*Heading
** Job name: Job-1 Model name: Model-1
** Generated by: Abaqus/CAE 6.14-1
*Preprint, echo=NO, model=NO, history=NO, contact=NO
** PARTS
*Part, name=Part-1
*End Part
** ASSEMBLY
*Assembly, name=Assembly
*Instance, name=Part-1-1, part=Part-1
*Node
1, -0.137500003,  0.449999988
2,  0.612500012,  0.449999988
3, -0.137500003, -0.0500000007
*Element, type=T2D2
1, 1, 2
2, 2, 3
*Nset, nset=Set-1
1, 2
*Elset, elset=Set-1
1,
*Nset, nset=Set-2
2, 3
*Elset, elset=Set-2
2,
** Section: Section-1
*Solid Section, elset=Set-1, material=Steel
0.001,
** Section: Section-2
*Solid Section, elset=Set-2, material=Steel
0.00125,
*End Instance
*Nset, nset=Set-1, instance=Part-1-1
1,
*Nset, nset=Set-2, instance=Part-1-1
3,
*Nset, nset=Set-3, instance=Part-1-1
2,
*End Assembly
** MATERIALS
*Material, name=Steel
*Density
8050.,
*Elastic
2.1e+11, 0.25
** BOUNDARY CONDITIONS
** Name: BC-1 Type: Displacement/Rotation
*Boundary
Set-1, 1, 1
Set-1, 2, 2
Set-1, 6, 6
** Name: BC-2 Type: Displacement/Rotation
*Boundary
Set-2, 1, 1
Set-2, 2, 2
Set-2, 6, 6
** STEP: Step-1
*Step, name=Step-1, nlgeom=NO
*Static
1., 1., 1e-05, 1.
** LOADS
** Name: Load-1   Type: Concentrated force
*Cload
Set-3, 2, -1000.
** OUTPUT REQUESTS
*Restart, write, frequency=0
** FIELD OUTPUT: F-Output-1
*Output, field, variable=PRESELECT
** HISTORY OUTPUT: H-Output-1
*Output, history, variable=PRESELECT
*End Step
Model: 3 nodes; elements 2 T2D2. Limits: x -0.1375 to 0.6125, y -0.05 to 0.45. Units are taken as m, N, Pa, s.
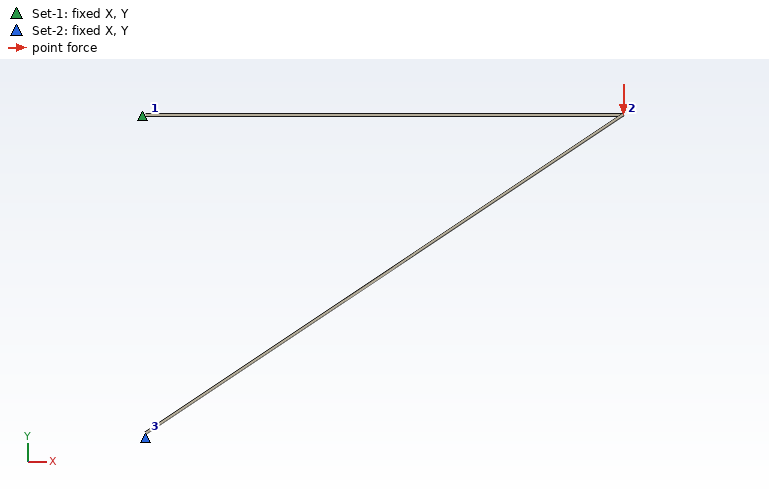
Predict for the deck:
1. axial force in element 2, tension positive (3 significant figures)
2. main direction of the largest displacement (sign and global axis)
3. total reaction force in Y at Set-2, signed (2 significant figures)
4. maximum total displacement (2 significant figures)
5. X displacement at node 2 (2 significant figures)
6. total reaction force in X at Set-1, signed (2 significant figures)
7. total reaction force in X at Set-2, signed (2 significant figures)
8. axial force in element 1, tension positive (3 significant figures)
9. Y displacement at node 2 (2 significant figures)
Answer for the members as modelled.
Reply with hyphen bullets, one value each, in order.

- -1800 N
- -Y
- 1000 N
- 2.0e-05 m
- 5.4e-06 m
- -1500 N
- 1500 N
- 1500 N
- -1.9e-05 m
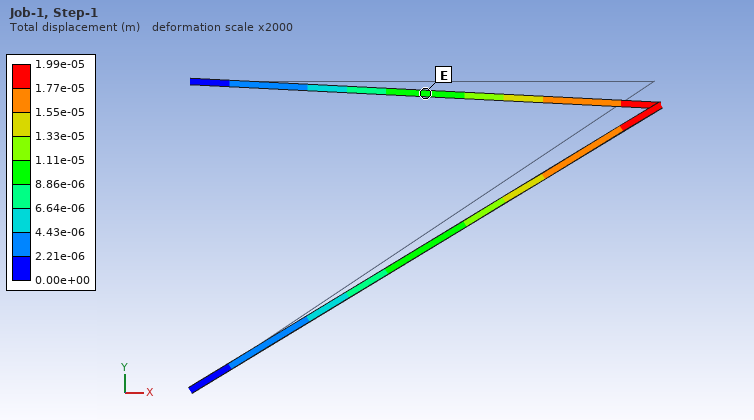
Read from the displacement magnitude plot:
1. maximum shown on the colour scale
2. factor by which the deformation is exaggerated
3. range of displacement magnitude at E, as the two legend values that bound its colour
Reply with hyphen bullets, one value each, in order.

- 1.99e-05 m
- 2000
- 8.86e-06 to 1.11e-05 m
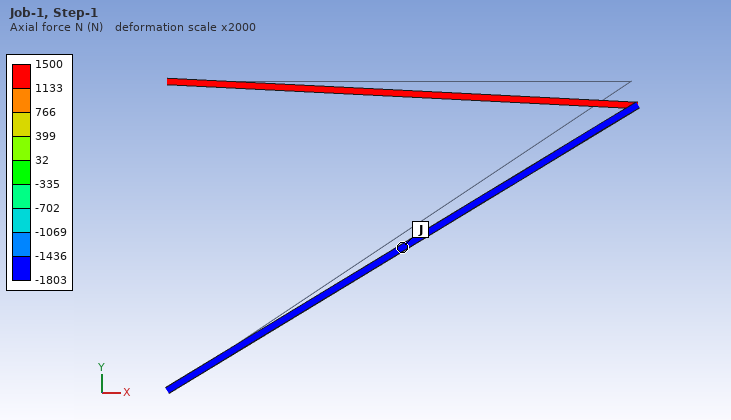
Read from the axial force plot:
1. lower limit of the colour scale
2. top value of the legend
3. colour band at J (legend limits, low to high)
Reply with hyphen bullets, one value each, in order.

- -1803 N
- 1500 N
- -1803 to -1436 N
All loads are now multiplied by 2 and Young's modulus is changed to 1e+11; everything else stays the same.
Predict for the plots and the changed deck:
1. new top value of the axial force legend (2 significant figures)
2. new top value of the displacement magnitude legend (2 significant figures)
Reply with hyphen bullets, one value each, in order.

- 3000 N
- 8.4e-05 m
